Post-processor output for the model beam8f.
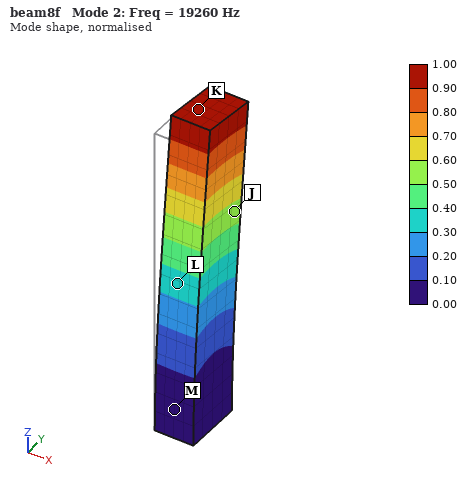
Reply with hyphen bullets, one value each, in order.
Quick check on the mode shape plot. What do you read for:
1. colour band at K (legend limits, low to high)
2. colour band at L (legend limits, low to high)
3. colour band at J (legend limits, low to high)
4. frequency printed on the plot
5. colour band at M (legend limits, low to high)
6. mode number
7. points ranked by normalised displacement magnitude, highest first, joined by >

- 0.90 to 1.00
- 0.30 to 0.40
- 0.50 to 0.60
- 19260 Hz
- 0.00 to 0.10
- 2
- K > J > L > M
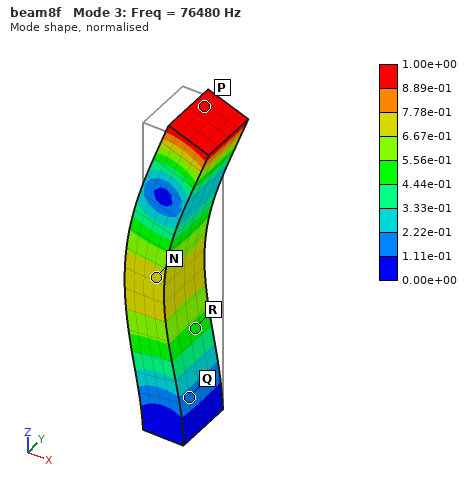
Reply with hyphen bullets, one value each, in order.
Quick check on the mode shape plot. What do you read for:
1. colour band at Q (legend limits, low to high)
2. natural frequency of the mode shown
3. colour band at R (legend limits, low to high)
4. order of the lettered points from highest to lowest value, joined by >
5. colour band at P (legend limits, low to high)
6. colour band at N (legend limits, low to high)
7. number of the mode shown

- 1.11e-01 to 2.22e-01
- 76480 Hz
- 4.44e-01 to 5.56e-01
- P > N > R > Q
- 8.89e-01 to 1.00e+00
- 6.67e-01 to 7.78e-01
- 3
